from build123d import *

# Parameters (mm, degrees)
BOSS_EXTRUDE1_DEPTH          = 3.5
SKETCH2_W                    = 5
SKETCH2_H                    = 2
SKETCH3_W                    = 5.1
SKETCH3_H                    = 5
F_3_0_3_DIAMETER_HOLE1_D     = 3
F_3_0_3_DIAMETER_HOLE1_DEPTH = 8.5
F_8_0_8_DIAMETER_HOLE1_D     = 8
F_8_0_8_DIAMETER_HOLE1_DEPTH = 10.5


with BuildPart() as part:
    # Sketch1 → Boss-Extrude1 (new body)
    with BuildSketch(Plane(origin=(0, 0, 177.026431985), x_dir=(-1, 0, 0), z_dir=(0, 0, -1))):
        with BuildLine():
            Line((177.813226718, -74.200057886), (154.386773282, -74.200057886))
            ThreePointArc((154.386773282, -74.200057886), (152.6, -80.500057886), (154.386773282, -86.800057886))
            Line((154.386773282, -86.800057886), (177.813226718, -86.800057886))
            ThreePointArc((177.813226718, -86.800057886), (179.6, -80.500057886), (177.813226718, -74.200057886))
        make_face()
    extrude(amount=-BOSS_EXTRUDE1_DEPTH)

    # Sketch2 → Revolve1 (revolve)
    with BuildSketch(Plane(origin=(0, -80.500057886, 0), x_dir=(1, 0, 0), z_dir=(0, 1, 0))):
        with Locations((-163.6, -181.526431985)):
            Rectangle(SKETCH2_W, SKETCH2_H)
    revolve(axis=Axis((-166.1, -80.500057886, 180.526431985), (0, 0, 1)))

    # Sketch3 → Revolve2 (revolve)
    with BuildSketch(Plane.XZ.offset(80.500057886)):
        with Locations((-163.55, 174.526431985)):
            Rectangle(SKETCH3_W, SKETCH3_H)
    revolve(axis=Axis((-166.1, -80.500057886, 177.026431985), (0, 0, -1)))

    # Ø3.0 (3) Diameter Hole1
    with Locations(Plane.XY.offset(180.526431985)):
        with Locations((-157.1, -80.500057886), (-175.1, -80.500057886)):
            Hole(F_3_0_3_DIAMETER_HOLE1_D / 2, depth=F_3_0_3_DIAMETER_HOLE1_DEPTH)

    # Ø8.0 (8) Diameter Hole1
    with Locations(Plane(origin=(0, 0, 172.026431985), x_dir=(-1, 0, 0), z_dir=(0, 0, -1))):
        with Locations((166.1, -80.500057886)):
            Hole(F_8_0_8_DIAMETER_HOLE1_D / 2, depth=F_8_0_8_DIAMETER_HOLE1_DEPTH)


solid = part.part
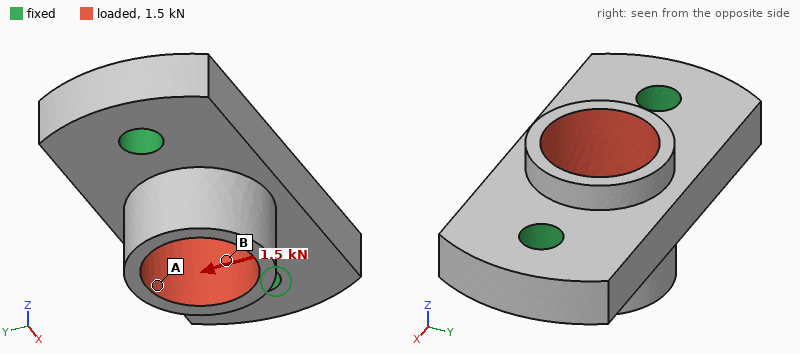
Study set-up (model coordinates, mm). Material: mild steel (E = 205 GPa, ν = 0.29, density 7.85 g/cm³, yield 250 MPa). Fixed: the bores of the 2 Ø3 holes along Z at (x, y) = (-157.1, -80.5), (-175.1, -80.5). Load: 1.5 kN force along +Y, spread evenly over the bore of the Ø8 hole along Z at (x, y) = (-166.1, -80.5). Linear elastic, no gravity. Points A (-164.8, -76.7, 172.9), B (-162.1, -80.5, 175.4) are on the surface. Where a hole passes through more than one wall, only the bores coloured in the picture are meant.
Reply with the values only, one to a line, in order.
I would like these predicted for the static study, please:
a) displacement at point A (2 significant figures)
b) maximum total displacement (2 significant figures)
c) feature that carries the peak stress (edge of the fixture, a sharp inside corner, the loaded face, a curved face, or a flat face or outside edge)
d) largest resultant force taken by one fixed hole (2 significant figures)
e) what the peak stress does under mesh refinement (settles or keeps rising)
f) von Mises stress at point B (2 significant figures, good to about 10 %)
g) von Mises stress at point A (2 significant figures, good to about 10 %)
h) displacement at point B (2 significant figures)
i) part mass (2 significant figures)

7.0 µm
8.1 µm
edge of the fixture
750 N
keeps rising
65 MPa
20 MPa
3.8 µm
8.9 g
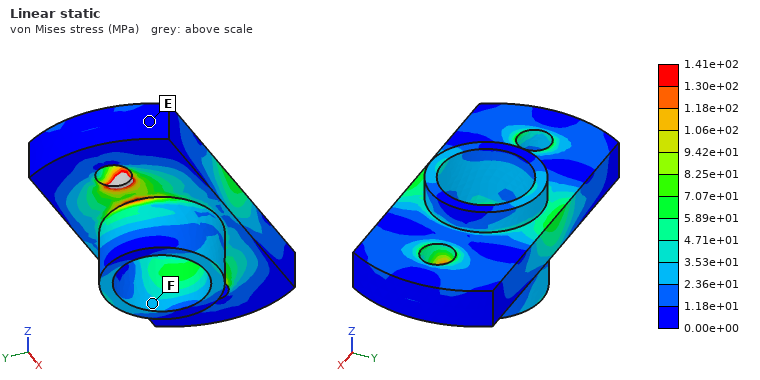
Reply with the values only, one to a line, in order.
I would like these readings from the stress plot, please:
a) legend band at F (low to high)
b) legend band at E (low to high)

2.36e+01 to 3.53e+01 MPa
0.00e+00 to 1.18e+01 MPa
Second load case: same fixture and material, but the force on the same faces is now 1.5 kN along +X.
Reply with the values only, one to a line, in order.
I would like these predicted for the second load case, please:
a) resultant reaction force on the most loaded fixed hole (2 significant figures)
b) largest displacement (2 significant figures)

770 N
3.7 µm
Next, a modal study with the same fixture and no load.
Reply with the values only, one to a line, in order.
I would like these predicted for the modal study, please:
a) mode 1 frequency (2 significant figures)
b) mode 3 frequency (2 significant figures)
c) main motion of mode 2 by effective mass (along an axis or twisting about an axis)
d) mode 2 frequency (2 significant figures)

34 kHz
57 kHz
along Z
42 kHz
